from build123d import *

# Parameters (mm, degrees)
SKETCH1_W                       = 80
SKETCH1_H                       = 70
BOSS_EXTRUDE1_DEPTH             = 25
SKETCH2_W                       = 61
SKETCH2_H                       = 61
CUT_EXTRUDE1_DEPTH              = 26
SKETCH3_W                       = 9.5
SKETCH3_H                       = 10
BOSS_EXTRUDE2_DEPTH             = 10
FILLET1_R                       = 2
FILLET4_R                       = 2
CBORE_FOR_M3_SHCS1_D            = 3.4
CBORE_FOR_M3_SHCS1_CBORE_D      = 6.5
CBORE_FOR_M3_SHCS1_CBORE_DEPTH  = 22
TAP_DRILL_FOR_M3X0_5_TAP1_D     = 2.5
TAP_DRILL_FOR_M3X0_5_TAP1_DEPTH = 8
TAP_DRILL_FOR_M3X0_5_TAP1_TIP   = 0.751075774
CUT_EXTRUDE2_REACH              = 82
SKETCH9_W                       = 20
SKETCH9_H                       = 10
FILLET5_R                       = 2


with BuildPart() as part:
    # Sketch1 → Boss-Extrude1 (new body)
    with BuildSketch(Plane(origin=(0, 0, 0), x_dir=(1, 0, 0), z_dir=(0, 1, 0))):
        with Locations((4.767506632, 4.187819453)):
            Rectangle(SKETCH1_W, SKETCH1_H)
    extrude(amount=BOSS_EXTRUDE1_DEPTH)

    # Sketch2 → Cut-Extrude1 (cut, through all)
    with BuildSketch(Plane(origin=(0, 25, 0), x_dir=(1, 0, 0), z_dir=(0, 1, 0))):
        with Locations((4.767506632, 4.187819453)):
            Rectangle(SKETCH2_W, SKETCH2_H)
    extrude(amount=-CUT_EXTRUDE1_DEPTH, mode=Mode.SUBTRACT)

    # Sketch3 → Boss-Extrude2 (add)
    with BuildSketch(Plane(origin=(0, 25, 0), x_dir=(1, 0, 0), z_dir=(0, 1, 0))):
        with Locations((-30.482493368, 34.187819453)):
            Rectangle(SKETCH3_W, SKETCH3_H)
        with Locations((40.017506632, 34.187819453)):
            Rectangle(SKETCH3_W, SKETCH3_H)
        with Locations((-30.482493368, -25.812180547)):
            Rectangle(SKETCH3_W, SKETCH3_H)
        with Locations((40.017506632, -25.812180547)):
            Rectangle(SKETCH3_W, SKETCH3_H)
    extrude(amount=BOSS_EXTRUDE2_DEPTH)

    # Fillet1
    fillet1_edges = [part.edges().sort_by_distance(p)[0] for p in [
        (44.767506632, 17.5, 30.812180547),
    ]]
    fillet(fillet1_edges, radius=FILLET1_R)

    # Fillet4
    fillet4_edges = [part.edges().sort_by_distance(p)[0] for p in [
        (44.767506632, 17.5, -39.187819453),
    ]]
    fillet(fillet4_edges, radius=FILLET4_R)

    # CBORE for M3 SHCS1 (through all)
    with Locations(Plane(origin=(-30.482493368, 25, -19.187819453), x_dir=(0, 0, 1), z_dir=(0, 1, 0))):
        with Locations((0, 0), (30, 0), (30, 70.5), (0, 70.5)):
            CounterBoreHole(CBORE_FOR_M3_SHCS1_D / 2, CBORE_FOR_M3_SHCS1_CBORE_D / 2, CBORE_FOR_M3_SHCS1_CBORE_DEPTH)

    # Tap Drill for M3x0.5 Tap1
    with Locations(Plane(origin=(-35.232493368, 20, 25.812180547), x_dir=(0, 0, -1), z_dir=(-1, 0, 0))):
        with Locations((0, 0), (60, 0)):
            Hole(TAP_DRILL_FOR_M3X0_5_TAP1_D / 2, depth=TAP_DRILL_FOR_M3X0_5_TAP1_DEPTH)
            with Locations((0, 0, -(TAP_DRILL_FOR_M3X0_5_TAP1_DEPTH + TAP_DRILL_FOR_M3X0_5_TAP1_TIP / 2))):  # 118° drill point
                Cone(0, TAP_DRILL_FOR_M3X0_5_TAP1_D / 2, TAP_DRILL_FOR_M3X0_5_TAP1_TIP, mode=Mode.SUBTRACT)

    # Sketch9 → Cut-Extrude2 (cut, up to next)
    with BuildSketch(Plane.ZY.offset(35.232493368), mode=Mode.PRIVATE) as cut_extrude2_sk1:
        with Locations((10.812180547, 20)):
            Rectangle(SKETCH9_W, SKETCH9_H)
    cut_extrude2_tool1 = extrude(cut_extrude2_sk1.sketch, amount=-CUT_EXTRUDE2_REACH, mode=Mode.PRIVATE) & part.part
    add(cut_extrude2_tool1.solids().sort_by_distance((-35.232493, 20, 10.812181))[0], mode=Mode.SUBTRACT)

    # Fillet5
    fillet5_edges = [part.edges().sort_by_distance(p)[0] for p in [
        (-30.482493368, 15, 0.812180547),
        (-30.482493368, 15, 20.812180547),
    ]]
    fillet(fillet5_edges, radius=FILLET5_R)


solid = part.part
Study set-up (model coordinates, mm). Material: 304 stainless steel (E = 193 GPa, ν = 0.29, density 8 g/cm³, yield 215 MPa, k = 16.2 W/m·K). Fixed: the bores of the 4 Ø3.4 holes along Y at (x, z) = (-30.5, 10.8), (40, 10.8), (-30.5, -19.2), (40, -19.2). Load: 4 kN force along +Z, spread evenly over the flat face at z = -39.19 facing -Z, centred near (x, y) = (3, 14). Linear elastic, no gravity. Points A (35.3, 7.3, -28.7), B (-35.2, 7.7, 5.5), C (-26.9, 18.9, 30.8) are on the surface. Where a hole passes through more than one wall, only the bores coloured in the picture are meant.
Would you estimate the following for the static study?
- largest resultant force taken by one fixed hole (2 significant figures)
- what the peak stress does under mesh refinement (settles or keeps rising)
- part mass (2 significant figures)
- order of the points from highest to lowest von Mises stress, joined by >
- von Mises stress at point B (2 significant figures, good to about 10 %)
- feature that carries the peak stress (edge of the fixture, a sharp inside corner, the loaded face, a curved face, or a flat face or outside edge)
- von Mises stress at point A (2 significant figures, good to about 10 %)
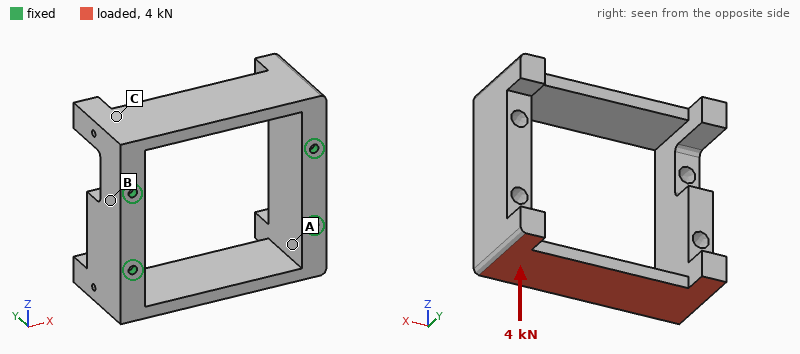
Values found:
1.6 kN
keeps rising
370 g
A > B > C
26 MPa
edge of the fixture
46 MPa
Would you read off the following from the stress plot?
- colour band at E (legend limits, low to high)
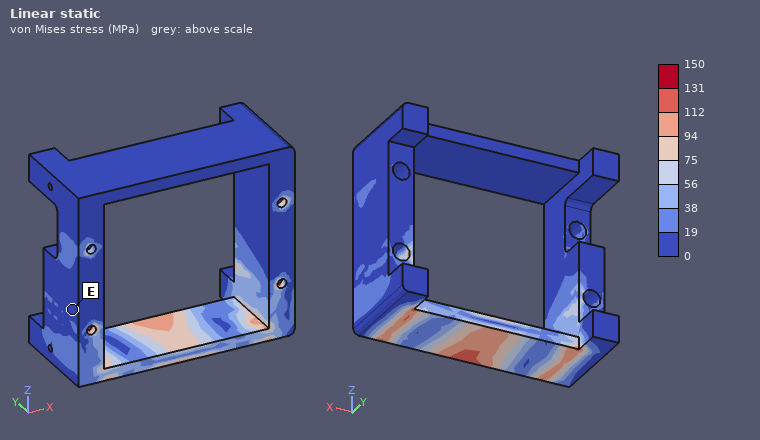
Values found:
0 to 19 MPa
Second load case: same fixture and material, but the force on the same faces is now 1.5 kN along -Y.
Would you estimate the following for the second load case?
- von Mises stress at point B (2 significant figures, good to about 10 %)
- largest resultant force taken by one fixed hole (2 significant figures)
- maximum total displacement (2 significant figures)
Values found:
12 MPa
1.3 kN
15 µm
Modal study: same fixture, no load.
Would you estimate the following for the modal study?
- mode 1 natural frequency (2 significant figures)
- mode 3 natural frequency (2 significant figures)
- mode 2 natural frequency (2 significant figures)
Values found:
4200 Hz
4600 Hz
4600 Hz
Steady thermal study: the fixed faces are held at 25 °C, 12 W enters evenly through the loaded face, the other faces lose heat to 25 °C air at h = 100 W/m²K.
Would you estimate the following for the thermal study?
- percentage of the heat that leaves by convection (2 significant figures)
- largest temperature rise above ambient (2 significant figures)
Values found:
83 %
31 K
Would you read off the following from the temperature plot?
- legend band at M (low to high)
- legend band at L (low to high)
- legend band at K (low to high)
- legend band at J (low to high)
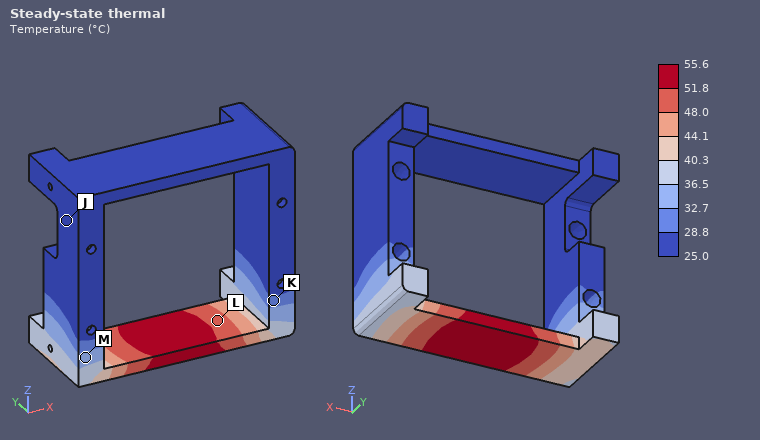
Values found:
32.7 to 36.5 °C
48.0 to 51.8 °C
28.8 to 32.7 °C
25.0 to 28.8 °C
